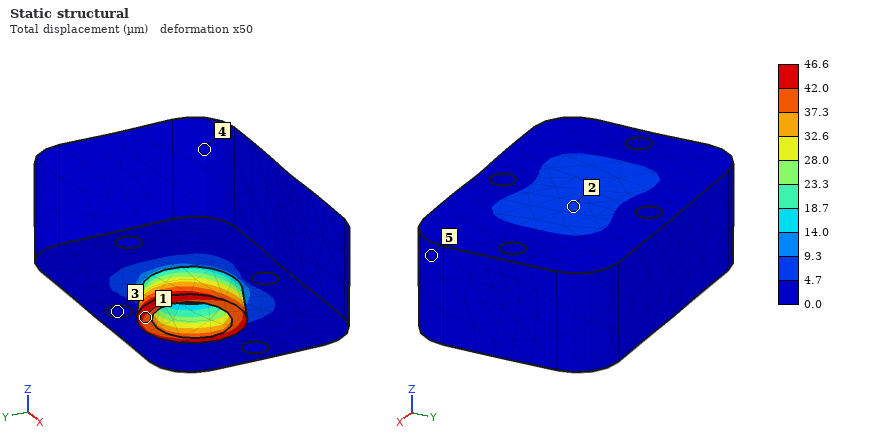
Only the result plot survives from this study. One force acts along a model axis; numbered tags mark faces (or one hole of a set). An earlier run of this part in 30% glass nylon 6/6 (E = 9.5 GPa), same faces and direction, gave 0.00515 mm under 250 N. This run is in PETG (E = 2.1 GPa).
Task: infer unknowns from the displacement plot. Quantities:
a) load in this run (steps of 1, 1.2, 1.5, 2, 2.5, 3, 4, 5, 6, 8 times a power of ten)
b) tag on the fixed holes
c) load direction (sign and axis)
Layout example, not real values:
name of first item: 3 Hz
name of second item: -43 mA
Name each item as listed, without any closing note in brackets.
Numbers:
load in this run: 500 N
tag on the fixed holes: 3
load direction: +Z
